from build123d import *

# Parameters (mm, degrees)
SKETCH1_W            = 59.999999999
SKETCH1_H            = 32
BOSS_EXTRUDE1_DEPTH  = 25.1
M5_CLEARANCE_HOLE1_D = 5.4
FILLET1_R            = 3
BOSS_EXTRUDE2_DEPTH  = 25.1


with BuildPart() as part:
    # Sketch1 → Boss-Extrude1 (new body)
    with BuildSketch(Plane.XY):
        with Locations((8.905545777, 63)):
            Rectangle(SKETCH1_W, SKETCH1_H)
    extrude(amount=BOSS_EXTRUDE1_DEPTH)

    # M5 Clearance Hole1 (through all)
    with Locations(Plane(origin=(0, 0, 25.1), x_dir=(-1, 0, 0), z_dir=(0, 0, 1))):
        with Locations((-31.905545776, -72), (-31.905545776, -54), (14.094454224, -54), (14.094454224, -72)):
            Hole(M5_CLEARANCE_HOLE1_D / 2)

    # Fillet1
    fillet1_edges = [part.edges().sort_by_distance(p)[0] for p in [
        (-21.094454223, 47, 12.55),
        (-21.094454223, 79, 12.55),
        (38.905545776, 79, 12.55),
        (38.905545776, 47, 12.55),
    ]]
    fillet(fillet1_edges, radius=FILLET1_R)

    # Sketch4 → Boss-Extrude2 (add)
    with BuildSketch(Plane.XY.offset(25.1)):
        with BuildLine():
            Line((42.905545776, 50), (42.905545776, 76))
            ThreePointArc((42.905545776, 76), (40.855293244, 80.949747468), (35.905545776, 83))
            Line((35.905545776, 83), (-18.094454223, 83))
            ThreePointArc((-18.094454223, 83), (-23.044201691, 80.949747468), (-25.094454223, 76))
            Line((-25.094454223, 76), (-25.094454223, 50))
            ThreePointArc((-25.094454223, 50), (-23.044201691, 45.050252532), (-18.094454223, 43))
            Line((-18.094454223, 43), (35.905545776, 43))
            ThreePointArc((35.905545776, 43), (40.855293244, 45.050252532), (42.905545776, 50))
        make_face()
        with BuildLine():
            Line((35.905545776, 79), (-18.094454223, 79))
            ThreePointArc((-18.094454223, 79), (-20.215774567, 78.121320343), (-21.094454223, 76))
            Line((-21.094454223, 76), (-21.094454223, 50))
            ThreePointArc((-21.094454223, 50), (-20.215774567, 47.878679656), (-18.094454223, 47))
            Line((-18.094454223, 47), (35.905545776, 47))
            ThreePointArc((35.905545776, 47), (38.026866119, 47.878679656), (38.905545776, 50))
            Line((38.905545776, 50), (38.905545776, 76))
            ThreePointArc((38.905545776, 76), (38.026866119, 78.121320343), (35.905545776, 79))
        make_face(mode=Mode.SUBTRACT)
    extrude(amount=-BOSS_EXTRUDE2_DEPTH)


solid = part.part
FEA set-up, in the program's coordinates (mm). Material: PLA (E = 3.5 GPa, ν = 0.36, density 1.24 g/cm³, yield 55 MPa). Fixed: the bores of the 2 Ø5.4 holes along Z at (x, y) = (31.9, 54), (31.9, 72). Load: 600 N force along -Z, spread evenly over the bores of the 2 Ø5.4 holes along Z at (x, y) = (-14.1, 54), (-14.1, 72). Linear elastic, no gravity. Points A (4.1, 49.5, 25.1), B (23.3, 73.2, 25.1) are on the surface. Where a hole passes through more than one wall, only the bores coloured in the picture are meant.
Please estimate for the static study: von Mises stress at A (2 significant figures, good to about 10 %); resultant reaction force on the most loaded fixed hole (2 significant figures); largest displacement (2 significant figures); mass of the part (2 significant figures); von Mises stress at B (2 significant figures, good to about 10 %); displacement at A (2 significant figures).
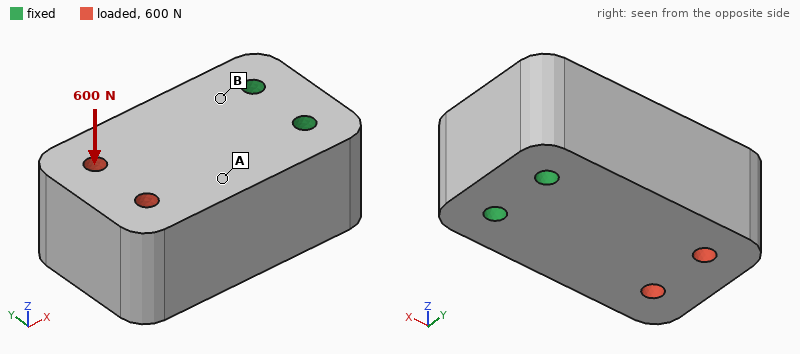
2.6 MPa
300 N
0.18 mm
80 g
6.2 MPa
0.076 mm
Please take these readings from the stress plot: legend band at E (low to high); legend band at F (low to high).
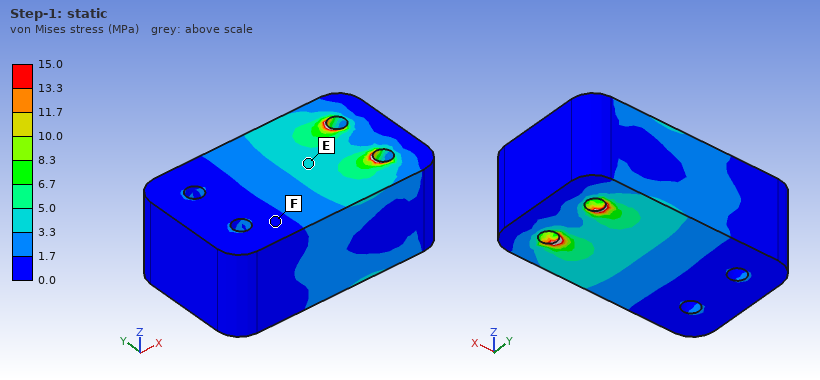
3.3 to 5.0 MPa
0.0 to 1.7 MPa
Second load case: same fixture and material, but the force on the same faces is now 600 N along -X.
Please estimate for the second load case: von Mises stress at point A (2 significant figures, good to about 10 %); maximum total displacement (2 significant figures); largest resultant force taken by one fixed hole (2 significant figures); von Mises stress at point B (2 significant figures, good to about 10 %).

0.57 MPa
9.8 µm
300 N
0.71 MPa
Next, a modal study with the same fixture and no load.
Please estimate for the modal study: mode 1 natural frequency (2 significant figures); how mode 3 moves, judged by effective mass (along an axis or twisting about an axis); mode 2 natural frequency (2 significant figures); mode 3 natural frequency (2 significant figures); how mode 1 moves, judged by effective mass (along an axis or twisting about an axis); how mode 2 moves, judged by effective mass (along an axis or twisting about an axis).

1900 Hz
twisting about X
2300 Hz
4000 Hz
along Z
along Y
